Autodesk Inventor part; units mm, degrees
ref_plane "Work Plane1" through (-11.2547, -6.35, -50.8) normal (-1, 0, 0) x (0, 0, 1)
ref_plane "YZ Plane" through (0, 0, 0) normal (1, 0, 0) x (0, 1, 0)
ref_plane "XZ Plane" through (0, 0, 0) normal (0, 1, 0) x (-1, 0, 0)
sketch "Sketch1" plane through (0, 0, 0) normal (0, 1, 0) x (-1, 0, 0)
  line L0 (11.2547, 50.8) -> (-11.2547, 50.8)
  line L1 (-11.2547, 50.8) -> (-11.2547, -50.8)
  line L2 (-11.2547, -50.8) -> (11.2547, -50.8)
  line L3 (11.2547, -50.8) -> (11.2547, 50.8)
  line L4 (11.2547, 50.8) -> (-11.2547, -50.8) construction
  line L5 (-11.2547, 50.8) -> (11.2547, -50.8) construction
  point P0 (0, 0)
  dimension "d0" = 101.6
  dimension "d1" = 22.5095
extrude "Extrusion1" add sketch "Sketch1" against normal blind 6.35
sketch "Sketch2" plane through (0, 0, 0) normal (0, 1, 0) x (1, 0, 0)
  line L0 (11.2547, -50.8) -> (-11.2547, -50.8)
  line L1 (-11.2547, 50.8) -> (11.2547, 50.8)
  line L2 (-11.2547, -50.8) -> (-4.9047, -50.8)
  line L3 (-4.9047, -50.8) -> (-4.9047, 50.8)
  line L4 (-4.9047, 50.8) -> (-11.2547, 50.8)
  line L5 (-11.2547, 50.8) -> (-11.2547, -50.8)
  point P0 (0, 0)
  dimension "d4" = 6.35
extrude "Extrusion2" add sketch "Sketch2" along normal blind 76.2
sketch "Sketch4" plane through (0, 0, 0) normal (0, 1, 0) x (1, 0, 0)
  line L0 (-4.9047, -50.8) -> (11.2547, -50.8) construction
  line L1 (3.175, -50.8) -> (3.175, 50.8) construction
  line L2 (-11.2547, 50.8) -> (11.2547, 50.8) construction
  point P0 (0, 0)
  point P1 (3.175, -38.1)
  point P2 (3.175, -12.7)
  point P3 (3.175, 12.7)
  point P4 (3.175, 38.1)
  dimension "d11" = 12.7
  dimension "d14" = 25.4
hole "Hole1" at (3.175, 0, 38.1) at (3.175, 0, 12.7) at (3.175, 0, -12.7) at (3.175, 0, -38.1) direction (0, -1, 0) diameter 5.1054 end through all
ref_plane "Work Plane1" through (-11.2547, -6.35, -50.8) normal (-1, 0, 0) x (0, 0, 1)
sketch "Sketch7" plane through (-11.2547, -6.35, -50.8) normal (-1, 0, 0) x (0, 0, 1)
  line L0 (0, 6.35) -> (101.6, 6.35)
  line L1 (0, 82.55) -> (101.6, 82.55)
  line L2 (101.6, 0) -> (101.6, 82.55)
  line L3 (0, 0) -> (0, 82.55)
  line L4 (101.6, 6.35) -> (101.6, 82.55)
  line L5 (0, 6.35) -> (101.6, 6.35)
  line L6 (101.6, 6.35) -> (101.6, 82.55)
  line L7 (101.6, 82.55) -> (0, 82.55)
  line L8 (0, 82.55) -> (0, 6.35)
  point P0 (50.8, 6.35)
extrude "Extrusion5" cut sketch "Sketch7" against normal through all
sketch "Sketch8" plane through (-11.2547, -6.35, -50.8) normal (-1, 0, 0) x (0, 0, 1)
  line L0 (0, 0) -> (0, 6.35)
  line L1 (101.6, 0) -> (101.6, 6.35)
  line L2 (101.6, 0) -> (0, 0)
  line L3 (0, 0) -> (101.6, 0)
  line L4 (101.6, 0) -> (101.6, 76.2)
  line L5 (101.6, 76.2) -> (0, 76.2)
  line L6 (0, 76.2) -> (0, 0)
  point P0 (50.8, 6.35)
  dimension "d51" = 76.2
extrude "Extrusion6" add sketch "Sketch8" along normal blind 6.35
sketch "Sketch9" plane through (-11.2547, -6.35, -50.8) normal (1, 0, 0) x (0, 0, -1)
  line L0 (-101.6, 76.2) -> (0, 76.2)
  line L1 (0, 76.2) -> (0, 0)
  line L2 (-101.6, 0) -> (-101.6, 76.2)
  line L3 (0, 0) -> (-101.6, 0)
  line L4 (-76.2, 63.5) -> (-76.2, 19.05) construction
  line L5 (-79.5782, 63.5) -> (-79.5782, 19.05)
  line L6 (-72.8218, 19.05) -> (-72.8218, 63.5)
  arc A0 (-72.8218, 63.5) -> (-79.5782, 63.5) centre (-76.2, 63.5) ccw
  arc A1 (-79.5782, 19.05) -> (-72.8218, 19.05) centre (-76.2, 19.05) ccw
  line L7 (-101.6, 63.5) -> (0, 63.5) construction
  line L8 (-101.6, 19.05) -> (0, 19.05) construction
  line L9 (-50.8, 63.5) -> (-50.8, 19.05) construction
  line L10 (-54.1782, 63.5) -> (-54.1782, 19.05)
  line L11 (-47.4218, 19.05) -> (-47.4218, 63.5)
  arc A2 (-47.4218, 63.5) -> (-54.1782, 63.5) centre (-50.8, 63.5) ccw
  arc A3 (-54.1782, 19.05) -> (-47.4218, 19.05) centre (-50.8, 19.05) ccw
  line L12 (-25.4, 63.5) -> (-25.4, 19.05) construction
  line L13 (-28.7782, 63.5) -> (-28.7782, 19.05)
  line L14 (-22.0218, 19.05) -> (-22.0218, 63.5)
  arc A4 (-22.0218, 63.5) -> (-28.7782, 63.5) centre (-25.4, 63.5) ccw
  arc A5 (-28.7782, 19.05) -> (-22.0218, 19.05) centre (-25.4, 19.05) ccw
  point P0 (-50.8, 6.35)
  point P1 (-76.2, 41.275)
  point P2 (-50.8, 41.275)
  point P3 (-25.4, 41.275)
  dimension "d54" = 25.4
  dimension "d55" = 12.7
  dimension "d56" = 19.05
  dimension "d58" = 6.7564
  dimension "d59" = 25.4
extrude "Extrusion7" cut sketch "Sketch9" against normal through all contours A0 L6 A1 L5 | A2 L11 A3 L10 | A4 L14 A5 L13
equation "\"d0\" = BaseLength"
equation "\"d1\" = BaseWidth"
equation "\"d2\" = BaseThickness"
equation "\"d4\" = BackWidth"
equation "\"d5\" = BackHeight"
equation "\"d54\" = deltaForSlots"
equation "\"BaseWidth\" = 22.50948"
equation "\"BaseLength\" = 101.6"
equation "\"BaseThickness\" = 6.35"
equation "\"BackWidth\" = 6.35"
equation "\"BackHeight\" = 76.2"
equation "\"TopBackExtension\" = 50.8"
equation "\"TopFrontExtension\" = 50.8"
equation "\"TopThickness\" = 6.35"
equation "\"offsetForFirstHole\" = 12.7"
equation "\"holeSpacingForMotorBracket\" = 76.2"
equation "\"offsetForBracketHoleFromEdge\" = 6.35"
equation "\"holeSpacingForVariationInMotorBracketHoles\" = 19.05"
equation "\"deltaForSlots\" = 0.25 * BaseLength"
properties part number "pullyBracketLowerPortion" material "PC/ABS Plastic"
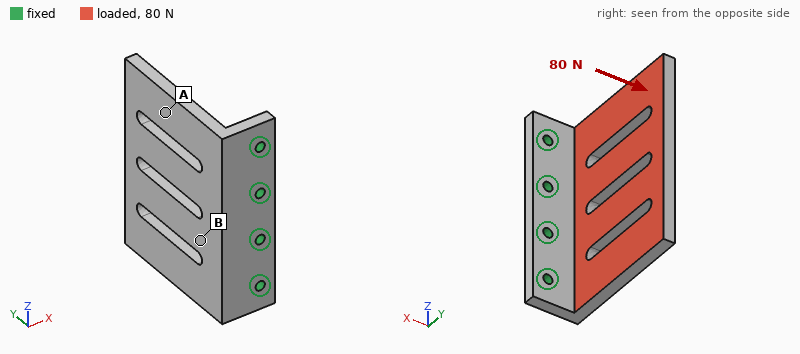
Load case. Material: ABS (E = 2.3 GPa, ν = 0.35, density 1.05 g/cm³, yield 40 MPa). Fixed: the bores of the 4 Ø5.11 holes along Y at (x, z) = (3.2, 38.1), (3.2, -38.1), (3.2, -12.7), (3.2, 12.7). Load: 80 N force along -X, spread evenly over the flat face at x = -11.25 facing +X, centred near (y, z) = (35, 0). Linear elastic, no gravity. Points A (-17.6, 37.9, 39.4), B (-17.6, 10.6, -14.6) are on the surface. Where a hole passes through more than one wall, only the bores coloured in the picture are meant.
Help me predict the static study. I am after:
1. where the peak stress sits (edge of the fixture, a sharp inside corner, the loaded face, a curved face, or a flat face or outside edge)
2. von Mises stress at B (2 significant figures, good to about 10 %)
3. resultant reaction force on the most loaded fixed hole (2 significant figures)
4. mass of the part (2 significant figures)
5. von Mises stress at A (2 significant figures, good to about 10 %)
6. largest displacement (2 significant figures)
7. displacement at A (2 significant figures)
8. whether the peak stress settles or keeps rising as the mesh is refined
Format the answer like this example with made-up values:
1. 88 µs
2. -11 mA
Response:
1. edge of the fixture
2. 3.2 MPa
3. 22 N
4. 60 g
5. 1.1 MPa
6. 1.6 mm
7. 0.76 mm
8. keeps rising
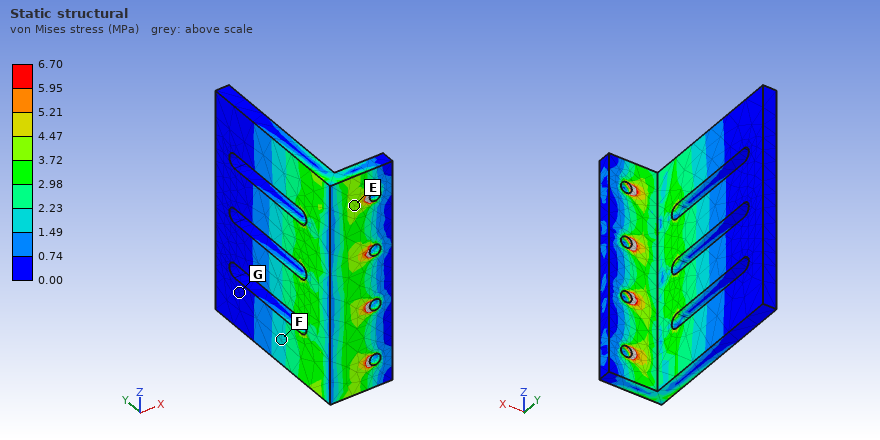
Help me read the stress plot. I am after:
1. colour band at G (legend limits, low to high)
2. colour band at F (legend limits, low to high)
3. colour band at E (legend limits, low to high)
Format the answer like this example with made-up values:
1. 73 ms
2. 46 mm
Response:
1. 0.00 to 0.74 MPa
2. 1.49 to 2.23 MPa
3. 3.72 to 4.47 MPa
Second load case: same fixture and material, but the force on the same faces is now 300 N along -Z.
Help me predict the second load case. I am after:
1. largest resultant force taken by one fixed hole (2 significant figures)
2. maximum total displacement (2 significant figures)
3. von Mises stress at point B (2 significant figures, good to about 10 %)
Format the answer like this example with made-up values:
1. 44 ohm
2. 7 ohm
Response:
1. 160 N
2. 0.74 mm
3. 1.7 MPa
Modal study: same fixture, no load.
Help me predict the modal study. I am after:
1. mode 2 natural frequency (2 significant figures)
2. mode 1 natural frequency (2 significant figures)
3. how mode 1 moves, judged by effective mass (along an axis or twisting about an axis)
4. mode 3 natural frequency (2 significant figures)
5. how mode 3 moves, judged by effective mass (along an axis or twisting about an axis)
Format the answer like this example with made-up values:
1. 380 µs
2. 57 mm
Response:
1. 420 Hz
2. 220 Hz
3. along X
4. 790 Hz
5. along Z
